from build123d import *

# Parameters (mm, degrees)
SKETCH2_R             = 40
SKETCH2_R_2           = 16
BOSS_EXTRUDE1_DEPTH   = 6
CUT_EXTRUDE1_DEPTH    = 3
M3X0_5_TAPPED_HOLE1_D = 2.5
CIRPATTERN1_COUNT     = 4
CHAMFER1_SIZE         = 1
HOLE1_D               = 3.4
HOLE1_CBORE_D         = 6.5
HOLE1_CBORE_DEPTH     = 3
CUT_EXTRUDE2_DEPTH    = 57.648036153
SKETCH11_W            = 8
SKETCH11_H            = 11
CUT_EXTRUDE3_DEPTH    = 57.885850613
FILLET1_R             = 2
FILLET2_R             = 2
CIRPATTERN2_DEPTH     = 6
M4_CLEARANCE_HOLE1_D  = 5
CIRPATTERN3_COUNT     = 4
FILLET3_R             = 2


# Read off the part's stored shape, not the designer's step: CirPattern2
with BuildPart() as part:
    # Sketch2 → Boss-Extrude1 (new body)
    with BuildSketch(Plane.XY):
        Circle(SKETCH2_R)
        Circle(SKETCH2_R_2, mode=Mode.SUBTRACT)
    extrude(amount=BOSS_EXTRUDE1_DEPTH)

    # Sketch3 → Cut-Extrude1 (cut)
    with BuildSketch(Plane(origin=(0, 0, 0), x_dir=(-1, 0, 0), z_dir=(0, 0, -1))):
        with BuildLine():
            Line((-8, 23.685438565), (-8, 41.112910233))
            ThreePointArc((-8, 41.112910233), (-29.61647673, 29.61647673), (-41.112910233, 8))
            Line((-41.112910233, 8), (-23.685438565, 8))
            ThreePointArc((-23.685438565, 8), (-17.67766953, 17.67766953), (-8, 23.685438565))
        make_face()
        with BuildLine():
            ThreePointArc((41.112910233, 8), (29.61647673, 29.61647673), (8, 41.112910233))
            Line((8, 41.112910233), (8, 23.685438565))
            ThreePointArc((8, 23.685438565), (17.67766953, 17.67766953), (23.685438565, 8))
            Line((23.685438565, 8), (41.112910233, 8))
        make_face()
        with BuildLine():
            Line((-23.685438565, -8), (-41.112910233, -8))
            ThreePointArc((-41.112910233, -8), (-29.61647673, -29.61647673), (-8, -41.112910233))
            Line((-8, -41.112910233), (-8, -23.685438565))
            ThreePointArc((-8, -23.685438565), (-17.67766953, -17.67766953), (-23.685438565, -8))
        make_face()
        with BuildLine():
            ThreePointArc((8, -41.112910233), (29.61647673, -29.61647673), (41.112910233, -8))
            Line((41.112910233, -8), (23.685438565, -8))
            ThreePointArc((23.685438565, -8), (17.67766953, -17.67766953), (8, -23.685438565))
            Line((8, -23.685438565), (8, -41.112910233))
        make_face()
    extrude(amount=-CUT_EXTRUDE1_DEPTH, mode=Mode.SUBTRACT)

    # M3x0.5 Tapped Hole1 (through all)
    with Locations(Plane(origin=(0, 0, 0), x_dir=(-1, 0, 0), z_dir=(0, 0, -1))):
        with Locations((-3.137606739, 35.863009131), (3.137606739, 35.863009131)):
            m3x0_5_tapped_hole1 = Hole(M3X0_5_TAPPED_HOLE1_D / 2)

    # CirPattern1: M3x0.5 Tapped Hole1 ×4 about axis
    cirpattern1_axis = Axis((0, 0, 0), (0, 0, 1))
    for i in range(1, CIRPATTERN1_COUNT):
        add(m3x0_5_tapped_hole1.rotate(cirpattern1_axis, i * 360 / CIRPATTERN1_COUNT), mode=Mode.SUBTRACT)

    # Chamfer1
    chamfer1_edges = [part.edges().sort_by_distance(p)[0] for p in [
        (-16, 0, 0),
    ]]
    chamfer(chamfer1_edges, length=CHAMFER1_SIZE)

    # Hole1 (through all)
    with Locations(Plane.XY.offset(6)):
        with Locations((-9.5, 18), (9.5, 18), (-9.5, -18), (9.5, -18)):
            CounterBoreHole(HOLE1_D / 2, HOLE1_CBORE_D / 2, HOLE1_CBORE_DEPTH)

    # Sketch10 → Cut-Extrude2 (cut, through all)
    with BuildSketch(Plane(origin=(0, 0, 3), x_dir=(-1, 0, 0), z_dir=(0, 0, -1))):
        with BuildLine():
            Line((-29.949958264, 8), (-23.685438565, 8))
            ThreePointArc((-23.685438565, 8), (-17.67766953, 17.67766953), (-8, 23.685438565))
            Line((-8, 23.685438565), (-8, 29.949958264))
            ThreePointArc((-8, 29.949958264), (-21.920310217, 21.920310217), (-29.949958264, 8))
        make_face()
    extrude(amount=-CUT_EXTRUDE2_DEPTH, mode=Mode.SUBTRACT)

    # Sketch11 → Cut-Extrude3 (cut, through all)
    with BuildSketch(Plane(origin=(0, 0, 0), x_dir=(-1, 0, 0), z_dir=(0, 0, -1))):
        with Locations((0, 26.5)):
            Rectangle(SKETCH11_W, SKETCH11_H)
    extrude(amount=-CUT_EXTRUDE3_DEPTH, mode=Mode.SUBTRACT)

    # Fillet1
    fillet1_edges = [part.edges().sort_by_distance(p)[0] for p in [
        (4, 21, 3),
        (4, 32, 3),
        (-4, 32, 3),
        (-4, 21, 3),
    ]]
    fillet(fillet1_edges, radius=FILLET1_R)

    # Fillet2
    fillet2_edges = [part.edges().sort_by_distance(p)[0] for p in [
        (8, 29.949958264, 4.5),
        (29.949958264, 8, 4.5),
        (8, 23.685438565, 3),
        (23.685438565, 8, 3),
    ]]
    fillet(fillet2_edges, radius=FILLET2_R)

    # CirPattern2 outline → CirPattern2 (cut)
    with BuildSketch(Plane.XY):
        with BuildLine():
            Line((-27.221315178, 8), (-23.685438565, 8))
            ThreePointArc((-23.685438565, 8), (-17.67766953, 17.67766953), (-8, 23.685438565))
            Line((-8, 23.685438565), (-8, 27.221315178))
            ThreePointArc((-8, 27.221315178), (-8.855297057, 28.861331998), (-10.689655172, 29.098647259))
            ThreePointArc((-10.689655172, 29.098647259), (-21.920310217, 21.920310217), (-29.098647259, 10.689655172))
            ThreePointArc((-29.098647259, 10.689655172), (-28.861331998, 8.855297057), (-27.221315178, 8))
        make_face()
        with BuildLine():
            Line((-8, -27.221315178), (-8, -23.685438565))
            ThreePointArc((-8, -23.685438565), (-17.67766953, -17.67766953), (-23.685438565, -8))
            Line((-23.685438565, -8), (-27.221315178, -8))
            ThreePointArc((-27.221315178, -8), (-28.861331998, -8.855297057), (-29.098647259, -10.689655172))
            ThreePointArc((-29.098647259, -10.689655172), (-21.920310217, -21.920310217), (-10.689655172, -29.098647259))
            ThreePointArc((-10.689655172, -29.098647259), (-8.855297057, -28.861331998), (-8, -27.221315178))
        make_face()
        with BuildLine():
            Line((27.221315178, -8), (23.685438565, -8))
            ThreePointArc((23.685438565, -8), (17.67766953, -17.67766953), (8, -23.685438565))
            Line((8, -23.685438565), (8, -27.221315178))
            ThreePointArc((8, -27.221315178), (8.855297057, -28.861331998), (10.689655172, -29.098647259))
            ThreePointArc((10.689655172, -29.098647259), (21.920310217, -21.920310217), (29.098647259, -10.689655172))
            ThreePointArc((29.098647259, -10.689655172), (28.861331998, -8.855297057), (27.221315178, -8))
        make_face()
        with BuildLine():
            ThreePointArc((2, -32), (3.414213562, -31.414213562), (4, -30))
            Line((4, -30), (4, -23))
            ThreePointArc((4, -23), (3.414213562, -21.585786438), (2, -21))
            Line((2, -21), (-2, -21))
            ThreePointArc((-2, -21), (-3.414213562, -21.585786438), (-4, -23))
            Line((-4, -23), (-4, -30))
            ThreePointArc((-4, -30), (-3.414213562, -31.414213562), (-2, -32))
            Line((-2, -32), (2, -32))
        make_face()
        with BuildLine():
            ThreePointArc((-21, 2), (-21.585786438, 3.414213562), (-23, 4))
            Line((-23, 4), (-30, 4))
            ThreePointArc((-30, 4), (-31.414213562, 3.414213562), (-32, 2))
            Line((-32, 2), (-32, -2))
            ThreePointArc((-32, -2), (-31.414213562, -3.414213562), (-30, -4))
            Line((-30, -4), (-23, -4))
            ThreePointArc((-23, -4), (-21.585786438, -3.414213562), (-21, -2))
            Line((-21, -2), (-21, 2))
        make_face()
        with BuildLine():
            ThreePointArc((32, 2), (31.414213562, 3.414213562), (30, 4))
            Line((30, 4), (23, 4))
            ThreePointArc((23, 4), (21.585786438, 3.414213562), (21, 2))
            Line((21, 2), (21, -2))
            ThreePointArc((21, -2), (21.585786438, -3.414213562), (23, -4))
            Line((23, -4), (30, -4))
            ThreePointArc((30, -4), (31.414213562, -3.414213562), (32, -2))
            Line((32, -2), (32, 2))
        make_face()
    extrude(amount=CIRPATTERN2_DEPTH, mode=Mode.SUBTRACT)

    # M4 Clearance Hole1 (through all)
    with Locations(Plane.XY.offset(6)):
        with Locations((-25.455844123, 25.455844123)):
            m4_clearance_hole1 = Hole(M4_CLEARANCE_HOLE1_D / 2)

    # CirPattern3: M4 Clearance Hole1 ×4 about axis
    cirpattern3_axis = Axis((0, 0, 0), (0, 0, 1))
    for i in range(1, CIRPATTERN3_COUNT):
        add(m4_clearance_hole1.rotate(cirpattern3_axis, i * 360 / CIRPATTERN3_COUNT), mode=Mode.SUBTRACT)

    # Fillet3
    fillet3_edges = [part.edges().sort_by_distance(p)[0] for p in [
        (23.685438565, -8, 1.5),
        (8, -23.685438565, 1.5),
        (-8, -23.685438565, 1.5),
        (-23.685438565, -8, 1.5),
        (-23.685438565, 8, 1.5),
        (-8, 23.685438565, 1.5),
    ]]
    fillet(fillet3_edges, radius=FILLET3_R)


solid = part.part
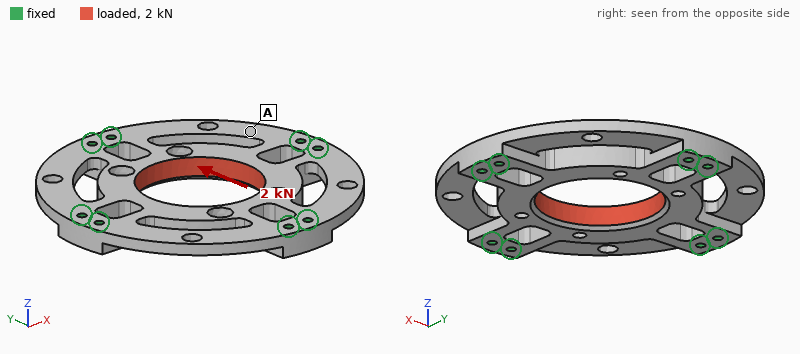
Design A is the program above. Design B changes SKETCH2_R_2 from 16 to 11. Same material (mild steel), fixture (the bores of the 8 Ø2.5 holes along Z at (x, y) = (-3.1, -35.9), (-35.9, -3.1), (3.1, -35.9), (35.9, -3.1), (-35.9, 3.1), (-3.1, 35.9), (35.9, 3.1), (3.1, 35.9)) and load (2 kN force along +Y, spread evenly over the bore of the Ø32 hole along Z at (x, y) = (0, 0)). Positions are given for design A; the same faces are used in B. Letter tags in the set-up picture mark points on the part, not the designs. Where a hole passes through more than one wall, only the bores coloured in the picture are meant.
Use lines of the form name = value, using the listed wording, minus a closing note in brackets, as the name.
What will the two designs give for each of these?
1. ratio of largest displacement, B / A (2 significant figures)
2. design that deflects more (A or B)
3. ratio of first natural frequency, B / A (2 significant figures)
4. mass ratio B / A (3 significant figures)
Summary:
ratio of largest displacement, B / A = 0.67
design that deflects more = A
ratio of first natural frequency, B / A = 0.88
mass ratio B / A = 1.18
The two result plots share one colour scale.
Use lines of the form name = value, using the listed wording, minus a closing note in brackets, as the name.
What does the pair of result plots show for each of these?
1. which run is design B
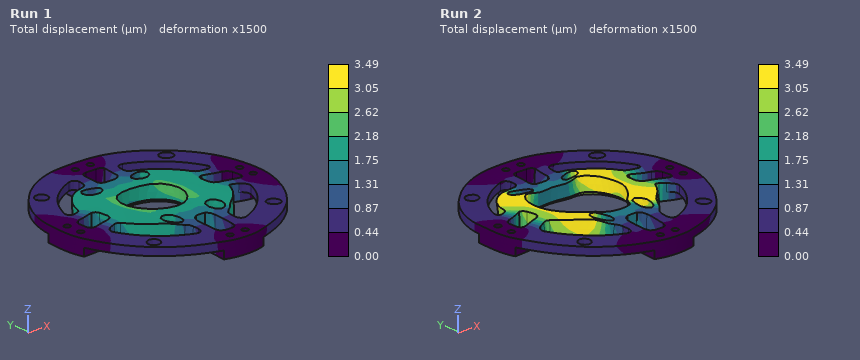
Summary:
which run is design B = Run 1
